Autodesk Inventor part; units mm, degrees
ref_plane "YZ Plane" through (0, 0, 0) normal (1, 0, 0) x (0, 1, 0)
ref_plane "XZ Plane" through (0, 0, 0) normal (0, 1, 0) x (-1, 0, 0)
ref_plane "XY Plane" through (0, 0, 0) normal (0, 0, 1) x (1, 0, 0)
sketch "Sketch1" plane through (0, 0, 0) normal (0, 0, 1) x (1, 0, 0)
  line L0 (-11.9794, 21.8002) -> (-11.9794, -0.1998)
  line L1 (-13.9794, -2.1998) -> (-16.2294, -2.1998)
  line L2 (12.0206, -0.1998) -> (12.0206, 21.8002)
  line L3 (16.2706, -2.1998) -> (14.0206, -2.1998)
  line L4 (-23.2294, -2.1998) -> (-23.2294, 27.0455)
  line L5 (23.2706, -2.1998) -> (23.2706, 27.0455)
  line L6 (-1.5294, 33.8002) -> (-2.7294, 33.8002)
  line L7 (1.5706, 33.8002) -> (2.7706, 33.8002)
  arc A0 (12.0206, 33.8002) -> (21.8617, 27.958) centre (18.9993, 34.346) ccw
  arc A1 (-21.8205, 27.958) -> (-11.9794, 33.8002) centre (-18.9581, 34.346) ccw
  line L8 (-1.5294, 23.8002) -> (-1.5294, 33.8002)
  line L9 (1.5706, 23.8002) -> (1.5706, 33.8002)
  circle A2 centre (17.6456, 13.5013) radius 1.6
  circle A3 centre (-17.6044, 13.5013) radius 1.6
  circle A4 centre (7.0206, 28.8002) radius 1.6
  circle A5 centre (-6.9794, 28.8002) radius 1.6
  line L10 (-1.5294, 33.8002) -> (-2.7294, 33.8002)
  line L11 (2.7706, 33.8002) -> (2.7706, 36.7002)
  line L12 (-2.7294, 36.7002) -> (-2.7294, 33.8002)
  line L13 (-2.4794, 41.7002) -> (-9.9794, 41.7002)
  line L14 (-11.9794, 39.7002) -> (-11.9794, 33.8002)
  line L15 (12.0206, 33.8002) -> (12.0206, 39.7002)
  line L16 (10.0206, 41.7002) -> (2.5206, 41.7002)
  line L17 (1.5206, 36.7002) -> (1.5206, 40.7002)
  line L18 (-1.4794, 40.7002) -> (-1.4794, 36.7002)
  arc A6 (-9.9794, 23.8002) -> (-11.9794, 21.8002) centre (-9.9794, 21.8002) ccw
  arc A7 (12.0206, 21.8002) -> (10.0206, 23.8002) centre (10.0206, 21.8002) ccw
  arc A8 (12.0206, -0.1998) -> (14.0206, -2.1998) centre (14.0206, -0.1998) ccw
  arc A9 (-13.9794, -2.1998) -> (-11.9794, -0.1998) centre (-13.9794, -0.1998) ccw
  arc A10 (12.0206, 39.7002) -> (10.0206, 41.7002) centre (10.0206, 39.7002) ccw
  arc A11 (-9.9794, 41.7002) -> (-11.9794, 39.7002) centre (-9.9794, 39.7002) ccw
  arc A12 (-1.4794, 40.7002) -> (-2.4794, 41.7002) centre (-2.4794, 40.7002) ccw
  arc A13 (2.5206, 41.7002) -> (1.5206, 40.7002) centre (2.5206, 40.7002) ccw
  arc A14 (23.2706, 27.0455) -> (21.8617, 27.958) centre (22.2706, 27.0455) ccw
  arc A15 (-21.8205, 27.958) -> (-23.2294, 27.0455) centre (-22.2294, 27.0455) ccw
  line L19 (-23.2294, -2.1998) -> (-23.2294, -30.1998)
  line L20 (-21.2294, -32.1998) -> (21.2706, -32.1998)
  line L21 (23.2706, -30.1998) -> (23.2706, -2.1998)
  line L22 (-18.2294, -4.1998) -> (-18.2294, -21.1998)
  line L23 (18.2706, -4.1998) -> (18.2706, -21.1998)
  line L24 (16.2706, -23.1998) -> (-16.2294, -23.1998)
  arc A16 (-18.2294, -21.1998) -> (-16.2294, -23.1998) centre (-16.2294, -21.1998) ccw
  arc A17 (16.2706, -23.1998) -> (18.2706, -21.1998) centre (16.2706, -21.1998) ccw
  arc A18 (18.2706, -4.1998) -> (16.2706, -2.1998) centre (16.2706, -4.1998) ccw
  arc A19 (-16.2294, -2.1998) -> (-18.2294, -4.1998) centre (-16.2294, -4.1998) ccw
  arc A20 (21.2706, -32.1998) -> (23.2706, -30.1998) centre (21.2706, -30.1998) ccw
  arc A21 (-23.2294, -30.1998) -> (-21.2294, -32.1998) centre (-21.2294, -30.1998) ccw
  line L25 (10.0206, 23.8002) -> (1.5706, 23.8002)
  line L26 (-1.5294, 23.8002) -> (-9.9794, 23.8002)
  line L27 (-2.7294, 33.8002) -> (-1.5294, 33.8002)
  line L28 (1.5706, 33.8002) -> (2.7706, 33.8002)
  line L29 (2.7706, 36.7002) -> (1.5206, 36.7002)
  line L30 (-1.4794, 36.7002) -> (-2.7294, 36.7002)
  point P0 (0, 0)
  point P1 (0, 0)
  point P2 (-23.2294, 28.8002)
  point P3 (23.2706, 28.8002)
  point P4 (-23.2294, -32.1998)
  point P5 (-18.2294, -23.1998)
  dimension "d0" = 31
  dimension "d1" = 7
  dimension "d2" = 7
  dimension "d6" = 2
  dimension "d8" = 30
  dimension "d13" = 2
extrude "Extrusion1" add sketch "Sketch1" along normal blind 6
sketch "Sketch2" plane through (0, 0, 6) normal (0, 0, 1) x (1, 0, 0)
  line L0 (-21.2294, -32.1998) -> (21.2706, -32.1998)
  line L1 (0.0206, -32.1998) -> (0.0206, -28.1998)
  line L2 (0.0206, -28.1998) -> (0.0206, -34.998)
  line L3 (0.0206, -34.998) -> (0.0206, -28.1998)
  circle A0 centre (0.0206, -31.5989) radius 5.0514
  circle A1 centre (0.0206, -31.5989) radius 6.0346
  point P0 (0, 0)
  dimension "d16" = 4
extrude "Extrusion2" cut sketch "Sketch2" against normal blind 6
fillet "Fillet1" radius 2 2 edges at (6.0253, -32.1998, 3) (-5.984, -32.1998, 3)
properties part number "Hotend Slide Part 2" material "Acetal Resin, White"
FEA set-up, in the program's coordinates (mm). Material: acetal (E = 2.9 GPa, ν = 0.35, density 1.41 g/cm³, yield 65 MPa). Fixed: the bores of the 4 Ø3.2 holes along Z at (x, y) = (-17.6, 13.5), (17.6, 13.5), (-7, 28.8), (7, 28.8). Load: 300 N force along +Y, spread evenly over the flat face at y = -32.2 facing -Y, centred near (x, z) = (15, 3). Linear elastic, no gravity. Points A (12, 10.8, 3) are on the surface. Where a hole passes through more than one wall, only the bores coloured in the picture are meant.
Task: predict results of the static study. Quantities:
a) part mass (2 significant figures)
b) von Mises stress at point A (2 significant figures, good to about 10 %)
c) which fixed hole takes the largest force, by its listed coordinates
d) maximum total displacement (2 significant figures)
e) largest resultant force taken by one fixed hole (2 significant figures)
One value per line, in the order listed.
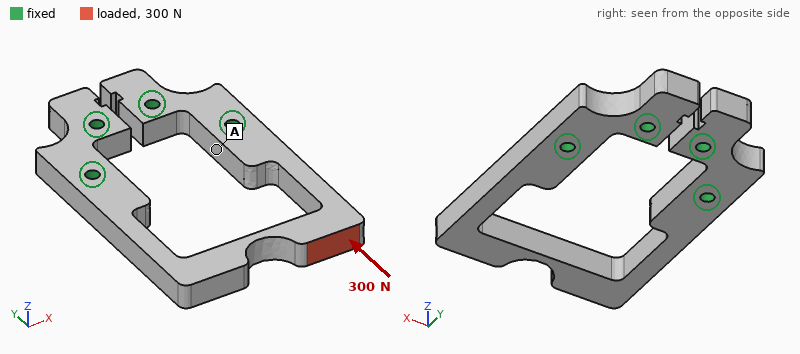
13 g
7.1 MPa
(17.6, 13.5)
0.75 mm
260 N
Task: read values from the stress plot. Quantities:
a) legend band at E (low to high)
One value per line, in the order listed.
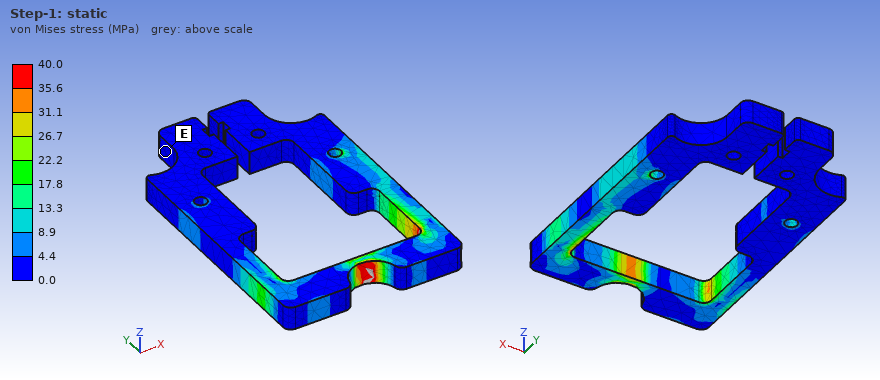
0.0 to 4.4 MPa
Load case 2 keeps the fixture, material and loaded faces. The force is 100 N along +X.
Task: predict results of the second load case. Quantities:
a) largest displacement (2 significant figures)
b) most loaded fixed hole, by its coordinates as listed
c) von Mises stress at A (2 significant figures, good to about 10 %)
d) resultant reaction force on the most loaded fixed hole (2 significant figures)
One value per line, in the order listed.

0.91 mm
(-17.6, 13.5)
7.9 MPa
140 N
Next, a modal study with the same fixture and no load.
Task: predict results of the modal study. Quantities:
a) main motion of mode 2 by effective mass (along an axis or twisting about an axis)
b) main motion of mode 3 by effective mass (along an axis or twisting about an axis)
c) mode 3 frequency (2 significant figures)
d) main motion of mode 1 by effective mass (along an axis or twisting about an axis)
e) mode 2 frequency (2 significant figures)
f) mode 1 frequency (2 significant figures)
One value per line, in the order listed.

twisting about Y
along X
990 Hz
along Z
900 Hz
500 Hz
